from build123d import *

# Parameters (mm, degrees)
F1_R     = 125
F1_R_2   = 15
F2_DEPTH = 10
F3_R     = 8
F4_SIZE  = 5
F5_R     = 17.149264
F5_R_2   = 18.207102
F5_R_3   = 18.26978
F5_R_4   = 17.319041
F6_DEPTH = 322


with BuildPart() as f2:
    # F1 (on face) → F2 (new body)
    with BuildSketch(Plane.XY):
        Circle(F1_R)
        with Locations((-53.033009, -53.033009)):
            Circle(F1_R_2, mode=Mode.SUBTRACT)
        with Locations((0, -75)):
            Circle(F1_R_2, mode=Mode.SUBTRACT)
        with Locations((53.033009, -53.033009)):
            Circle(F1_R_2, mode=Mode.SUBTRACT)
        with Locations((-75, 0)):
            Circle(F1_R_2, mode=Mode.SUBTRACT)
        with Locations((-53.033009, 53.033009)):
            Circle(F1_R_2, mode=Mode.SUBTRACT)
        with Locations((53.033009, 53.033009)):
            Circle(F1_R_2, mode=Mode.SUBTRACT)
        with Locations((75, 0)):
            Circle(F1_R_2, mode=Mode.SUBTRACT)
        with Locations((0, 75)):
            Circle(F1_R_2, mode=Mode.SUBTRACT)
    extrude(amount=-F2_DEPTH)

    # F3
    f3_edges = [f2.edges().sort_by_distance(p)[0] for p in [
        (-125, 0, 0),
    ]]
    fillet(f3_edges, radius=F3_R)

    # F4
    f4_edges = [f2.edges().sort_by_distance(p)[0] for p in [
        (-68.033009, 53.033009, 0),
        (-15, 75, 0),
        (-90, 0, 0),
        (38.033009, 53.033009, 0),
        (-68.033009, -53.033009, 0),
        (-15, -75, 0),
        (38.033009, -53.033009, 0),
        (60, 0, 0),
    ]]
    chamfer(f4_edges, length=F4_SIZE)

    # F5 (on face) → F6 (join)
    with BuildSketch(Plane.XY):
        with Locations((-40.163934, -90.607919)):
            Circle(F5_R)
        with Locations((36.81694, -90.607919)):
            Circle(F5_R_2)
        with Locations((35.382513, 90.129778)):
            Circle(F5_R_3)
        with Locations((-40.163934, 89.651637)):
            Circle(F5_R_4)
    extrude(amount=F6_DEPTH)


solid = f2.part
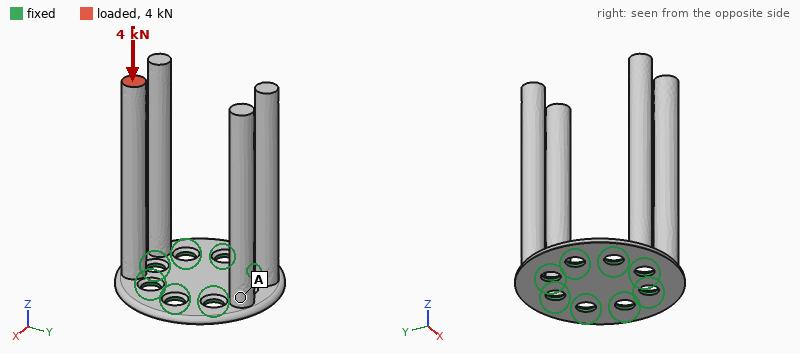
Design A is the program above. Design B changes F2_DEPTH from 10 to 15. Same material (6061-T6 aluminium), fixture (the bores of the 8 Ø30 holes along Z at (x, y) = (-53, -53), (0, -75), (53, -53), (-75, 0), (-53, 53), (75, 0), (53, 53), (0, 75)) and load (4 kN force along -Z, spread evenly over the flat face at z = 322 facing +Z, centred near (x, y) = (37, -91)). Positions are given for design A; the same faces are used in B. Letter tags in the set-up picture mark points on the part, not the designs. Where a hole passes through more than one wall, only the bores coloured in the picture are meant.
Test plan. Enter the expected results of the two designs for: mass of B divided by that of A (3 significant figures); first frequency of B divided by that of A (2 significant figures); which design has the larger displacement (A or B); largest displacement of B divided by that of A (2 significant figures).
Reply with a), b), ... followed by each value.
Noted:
a) 1.13
b) 1.3
c) A
d) 0.34
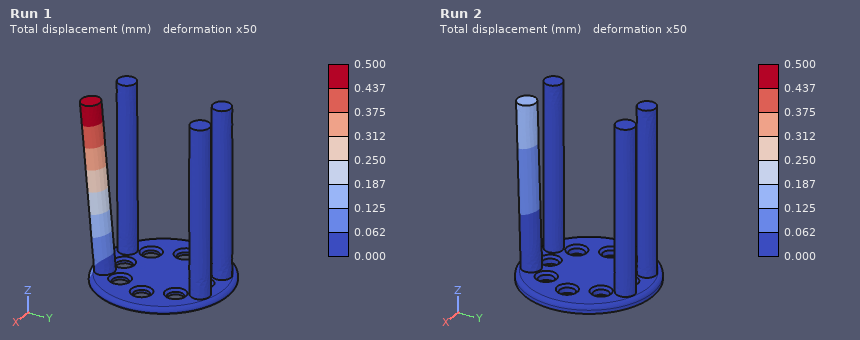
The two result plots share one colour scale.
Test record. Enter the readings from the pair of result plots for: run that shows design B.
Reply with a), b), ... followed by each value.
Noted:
a) Run 2
